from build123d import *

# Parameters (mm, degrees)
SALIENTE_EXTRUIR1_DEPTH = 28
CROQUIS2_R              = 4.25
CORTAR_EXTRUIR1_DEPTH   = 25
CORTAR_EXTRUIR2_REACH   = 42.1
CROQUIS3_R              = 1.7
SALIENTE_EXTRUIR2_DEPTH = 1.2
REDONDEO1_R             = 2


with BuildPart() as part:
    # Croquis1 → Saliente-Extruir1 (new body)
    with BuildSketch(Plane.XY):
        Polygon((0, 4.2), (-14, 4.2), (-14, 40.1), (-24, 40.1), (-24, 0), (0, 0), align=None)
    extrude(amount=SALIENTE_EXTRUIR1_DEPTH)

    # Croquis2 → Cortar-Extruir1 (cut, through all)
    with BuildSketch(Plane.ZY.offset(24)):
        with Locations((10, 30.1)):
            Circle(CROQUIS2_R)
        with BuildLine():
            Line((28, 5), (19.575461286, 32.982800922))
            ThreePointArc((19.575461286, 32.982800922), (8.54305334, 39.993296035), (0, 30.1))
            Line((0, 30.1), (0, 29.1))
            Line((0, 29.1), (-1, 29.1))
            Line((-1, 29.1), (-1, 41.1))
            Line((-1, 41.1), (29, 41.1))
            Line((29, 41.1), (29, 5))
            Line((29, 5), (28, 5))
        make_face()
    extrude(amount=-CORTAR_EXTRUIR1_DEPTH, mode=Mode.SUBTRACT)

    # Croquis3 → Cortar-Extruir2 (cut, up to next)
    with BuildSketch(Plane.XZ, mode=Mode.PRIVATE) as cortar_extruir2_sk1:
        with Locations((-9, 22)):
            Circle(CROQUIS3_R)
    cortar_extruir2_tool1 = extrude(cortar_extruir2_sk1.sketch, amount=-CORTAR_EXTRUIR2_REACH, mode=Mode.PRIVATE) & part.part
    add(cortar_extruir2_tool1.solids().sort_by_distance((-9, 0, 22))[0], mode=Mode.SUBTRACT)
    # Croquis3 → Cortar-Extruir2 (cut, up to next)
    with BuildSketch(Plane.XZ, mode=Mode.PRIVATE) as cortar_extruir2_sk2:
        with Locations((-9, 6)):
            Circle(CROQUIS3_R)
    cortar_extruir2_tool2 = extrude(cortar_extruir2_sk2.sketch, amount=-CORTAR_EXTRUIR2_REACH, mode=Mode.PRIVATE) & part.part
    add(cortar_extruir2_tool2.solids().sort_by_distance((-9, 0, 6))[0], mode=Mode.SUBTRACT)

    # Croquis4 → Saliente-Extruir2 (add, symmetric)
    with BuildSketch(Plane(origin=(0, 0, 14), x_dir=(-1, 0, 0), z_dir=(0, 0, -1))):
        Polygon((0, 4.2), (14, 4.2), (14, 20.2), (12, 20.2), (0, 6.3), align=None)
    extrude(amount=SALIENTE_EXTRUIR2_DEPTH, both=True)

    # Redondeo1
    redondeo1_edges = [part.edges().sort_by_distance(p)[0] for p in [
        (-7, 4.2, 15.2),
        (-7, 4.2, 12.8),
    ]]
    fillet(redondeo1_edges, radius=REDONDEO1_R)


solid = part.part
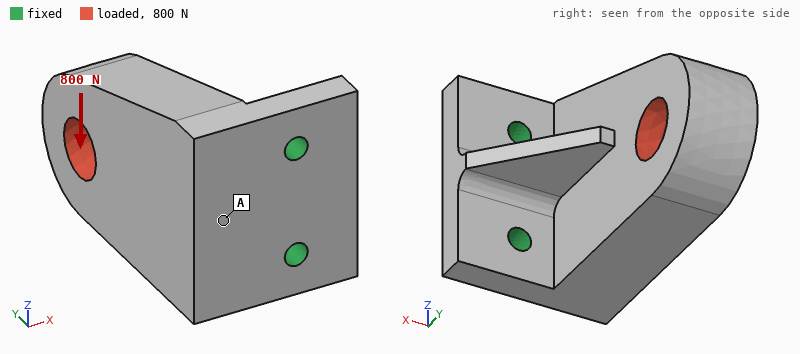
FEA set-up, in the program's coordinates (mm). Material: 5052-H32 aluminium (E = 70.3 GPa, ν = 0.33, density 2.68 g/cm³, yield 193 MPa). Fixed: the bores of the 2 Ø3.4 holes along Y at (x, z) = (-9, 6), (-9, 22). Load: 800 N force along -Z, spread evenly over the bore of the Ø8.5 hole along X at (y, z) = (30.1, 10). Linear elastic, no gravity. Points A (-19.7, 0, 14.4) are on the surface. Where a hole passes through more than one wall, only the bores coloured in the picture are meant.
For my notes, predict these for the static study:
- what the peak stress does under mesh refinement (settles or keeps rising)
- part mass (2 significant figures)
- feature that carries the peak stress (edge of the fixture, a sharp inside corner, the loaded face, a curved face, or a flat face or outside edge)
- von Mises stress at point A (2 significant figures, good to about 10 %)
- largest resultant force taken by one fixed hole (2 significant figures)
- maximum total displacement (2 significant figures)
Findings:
keeps rising
28 g
edge of the fixture
19 MPa
1.4 kN
77 µm
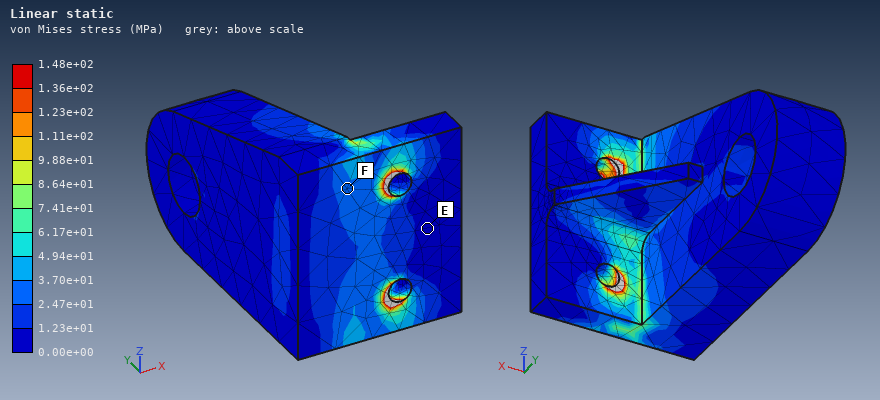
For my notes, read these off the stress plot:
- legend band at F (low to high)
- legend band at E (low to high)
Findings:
2.47e+01 to 3.70e+01 MPa
0.00e+00 to 1.23e+01 MPa
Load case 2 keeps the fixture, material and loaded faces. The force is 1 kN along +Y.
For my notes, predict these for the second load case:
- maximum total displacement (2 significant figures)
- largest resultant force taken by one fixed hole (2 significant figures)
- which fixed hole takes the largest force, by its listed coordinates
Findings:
89 µm
720 N
(-9, 6)
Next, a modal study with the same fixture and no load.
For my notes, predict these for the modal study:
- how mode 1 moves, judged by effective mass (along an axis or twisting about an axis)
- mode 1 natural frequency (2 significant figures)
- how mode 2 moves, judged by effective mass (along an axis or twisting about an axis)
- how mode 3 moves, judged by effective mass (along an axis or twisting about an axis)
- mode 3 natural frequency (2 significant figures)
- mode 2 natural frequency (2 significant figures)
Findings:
along X
3100 Hz
along Z
along Y
14 kHz
5800 Hz
